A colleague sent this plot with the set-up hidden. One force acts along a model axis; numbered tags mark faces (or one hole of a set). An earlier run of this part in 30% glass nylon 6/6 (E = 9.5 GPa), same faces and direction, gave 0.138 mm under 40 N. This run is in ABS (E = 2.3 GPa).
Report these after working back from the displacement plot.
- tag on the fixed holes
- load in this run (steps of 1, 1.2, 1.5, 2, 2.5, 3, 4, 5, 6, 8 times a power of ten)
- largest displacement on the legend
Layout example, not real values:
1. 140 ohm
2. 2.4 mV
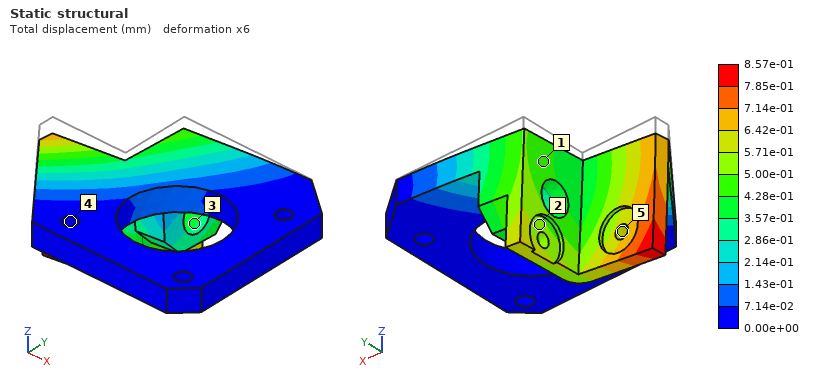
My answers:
1. 4
2. 60 N
3. 8.57e-01 mm
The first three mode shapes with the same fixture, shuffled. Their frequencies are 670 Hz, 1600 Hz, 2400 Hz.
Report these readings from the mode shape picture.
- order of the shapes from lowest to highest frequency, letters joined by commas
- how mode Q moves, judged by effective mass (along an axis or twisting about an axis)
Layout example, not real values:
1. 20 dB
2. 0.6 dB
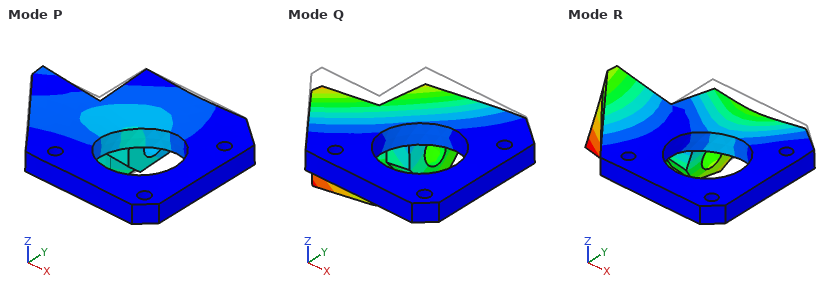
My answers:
1. Q, R, P
2. along Z
